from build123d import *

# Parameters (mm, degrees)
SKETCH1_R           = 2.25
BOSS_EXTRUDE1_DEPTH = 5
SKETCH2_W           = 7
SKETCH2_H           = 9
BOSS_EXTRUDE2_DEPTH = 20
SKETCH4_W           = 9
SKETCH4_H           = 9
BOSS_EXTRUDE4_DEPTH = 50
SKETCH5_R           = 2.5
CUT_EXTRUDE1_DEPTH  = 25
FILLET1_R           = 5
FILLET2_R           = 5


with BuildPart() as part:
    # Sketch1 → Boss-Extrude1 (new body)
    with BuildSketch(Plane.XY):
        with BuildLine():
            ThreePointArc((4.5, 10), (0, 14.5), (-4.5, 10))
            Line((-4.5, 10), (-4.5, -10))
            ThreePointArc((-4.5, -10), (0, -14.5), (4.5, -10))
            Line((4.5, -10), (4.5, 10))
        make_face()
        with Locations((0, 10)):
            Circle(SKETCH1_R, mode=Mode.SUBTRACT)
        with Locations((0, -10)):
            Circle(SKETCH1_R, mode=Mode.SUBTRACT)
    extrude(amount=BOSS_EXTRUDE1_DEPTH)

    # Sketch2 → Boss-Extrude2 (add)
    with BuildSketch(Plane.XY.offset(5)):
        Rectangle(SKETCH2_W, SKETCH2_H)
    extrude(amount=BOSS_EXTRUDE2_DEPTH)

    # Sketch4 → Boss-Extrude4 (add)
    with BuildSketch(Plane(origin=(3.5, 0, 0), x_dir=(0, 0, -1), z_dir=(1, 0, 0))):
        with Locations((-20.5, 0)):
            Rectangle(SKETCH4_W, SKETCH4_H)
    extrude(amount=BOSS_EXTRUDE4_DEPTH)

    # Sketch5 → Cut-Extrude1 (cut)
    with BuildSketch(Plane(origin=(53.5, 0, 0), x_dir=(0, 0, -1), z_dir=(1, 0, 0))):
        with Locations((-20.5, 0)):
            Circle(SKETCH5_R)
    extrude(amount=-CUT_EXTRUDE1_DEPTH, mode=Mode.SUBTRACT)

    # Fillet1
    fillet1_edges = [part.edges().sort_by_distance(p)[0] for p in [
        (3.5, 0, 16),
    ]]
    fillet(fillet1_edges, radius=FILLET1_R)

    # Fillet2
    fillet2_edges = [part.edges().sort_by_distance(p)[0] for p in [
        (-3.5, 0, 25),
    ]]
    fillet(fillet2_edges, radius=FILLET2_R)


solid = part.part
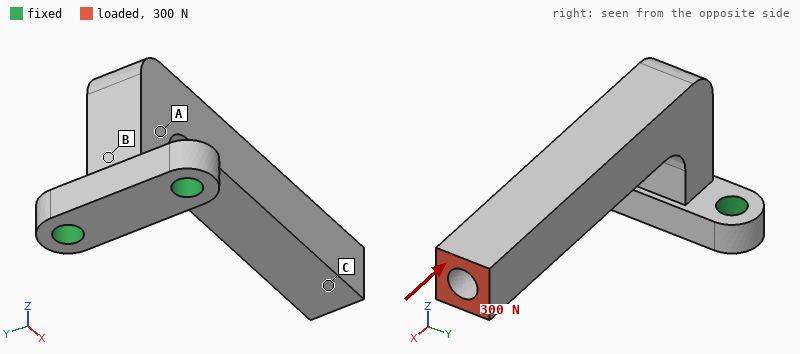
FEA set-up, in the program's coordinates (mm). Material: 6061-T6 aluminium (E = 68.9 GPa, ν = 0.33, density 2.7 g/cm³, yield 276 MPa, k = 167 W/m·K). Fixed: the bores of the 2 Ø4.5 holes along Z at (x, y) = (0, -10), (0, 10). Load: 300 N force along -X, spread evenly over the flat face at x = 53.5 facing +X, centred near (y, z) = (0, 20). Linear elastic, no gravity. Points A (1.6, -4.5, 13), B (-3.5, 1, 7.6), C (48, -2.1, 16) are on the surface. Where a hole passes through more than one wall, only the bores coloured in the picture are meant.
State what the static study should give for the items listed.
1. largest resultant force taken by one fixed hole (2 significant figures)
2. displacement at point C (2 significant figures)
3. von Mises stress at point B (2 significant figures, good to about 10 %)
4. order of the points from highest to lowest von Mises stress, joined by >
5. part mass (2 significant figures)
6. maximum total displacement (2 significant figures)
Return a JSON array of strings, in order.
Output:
["150 N", "0.21 mm", "48 MPa", "B > A > C", "16 g", "0.24 mm"]
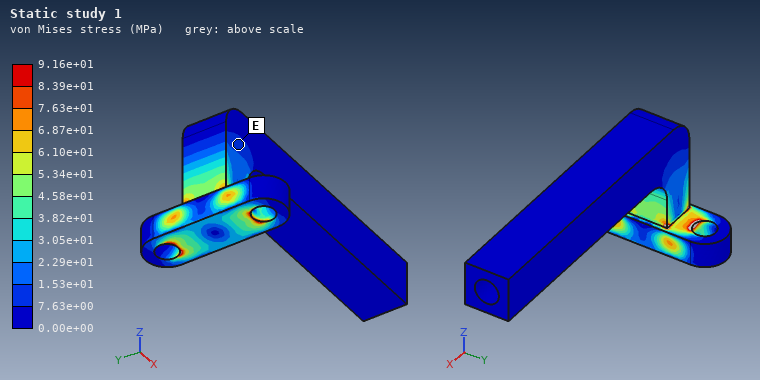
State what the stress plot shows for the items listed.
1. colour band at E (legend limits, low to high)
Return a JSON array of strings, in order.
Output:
["7.63e+00 to 1.53e+01 MPa"]
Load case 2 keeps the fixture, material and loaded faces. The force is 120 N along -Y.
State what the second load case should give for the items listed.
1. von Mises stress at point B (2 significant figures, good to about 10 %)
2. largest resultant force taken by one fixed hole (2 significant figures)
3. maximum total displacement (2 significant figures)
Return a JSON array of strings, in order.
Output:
["96 MPa", "410 N", "0.46 mm"]
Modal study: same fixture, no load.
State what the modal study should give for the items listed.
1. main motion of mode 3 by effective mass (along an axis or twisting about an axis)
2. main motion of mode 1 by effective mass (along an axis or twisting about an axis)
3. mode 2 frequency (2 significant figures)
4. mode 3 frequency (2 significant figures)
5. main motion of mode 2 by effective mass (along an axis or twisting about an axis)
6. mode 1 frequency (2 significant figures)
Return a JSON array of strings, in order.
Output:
["along X", "along Z", "1500 Hz", "5700 Hz", "along Y", "1400 Hz"]
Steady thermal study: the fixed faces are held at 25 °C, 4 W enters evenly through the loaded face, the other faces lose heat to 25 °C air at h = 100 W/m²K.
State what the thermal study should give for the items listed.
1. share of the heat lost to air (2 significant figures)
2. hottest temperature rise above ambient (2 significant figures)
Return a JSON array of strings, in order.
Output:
["53 %", "15 K"]
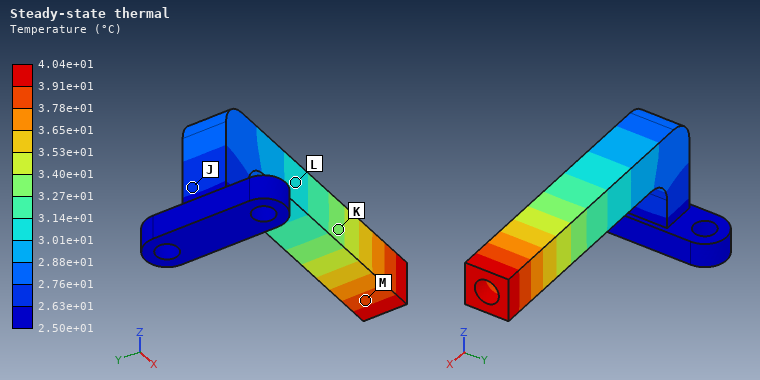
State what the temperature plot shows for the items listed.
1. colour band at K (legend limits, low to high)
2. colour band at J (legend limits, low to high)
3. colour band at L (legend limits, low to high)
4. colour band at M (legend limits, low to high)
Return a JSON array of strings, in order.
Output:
["3.27e+01 to 3.40e+01 °C", "2.63e+01 to 2.76e+01 °C", "3.01e+01 to 3.14e+01 °C", "3.78e+01 to 3.91e+01 °C"]
